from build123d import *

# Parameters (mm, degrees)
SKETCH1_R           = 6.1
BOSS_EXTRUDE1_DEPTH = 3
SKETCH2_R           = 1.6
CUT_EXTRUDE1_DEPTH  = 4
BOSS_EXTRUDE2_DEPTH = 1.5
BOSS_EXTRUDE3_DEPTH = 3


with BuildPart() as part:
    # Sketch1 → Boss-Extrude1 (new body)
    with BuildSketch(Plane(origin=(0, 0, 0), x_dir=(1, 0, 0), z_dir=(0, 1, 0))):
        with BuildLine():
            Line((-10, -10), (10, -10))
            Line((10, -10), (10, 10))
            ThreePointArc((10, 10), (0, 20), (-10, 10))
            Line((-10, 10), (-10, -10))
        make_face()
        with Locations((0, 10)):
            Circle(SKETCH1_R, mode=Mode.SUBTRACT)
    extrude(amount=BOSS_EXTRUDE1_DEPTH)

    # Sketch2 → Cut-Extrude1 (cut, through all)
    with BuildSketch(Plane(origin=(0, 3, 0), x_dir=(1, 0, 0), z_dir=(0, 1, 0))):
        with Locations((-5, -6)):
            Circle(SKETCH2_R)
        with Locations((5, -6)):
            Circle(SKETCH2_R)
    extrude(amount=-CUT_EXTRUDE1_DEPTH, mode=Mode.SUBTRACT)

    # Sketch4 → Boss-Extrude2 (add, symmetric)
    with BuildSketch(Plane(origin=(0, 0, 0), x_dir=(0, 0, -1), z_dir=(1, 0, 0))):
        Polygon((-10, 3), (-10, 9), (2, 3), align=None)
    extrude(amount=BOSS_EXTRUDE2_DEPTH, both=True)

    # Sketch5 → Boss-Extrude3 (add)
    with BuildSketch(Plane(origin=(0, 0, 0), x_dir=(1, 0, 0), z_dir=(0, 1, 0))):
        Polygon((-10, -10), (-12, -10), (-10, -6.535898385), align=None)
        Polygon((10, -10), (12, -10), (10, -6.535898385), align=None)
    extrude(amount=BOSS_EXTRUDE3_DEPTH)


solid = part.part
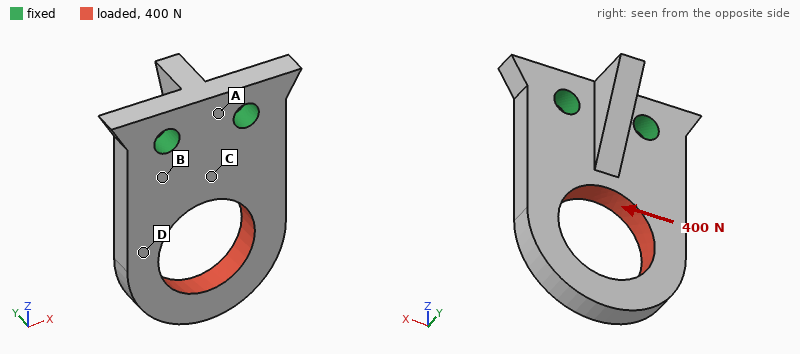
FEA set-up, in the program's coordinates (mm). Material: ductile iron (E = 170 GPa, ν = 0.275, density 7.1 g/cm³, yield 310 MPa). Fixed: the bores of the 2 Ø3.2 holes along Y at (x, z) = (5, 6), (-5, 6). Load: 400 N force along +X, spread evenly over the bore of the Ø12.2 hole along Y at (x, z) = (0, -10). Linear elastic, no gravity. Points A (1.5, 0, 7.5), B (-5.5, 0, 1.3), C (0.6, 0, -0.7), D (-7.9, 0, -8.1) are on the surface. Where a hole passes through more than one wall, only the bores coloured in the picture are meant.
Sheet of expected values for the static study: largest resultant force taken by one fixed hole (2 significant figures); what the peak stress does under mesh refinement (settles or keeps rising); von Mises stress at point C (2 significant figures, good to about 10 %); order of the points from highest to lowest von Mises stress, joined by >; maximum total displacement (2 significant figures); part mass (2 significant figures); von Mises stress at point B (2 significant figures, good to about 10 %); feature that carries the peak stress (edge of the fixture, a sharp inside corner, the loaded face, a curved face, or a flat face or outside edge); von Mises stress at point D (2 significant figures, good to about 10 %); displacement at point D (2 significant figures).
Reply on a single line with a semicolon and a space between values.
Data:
530 N; keeps rising; 34 MPa; C > D > B > A; 12 µm; 9.9 g; 12 MPa; edge of the fixture; 24 MPa; 5.6 µm
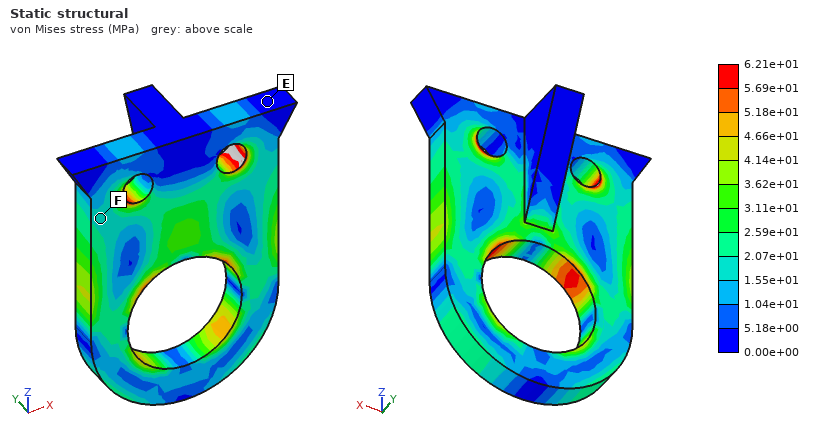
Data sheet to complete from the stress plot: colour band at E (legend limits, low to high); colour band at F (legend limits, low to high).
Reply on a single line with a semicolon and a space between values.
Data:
0.00e+00 to 5.18e+00 MPa; 1.55e+01 to 2.07e+01 MPa
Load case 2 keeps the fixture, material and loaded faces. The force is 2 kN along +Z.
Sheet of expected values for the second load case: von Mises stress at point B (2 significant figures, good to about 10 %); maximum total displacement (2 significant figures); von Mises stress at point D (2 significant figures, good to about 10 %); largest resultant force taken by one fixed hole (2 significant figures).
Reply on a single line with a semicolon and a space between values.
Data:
48 MPa; 12 µm; 57 MPa; 1.0 kN
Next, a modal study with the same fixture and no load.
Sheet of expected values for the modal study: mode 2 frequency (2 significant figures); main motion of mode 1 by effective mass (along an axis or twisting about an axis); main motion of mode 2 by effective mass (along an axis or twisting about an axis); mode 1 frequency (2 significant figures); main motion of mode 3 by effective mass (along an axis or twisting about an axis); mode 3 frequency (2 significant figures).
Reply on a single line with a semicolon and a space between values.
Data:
11 kHz; along Y; twisting about Z; 4800 Hz; along X; 15 kHz
